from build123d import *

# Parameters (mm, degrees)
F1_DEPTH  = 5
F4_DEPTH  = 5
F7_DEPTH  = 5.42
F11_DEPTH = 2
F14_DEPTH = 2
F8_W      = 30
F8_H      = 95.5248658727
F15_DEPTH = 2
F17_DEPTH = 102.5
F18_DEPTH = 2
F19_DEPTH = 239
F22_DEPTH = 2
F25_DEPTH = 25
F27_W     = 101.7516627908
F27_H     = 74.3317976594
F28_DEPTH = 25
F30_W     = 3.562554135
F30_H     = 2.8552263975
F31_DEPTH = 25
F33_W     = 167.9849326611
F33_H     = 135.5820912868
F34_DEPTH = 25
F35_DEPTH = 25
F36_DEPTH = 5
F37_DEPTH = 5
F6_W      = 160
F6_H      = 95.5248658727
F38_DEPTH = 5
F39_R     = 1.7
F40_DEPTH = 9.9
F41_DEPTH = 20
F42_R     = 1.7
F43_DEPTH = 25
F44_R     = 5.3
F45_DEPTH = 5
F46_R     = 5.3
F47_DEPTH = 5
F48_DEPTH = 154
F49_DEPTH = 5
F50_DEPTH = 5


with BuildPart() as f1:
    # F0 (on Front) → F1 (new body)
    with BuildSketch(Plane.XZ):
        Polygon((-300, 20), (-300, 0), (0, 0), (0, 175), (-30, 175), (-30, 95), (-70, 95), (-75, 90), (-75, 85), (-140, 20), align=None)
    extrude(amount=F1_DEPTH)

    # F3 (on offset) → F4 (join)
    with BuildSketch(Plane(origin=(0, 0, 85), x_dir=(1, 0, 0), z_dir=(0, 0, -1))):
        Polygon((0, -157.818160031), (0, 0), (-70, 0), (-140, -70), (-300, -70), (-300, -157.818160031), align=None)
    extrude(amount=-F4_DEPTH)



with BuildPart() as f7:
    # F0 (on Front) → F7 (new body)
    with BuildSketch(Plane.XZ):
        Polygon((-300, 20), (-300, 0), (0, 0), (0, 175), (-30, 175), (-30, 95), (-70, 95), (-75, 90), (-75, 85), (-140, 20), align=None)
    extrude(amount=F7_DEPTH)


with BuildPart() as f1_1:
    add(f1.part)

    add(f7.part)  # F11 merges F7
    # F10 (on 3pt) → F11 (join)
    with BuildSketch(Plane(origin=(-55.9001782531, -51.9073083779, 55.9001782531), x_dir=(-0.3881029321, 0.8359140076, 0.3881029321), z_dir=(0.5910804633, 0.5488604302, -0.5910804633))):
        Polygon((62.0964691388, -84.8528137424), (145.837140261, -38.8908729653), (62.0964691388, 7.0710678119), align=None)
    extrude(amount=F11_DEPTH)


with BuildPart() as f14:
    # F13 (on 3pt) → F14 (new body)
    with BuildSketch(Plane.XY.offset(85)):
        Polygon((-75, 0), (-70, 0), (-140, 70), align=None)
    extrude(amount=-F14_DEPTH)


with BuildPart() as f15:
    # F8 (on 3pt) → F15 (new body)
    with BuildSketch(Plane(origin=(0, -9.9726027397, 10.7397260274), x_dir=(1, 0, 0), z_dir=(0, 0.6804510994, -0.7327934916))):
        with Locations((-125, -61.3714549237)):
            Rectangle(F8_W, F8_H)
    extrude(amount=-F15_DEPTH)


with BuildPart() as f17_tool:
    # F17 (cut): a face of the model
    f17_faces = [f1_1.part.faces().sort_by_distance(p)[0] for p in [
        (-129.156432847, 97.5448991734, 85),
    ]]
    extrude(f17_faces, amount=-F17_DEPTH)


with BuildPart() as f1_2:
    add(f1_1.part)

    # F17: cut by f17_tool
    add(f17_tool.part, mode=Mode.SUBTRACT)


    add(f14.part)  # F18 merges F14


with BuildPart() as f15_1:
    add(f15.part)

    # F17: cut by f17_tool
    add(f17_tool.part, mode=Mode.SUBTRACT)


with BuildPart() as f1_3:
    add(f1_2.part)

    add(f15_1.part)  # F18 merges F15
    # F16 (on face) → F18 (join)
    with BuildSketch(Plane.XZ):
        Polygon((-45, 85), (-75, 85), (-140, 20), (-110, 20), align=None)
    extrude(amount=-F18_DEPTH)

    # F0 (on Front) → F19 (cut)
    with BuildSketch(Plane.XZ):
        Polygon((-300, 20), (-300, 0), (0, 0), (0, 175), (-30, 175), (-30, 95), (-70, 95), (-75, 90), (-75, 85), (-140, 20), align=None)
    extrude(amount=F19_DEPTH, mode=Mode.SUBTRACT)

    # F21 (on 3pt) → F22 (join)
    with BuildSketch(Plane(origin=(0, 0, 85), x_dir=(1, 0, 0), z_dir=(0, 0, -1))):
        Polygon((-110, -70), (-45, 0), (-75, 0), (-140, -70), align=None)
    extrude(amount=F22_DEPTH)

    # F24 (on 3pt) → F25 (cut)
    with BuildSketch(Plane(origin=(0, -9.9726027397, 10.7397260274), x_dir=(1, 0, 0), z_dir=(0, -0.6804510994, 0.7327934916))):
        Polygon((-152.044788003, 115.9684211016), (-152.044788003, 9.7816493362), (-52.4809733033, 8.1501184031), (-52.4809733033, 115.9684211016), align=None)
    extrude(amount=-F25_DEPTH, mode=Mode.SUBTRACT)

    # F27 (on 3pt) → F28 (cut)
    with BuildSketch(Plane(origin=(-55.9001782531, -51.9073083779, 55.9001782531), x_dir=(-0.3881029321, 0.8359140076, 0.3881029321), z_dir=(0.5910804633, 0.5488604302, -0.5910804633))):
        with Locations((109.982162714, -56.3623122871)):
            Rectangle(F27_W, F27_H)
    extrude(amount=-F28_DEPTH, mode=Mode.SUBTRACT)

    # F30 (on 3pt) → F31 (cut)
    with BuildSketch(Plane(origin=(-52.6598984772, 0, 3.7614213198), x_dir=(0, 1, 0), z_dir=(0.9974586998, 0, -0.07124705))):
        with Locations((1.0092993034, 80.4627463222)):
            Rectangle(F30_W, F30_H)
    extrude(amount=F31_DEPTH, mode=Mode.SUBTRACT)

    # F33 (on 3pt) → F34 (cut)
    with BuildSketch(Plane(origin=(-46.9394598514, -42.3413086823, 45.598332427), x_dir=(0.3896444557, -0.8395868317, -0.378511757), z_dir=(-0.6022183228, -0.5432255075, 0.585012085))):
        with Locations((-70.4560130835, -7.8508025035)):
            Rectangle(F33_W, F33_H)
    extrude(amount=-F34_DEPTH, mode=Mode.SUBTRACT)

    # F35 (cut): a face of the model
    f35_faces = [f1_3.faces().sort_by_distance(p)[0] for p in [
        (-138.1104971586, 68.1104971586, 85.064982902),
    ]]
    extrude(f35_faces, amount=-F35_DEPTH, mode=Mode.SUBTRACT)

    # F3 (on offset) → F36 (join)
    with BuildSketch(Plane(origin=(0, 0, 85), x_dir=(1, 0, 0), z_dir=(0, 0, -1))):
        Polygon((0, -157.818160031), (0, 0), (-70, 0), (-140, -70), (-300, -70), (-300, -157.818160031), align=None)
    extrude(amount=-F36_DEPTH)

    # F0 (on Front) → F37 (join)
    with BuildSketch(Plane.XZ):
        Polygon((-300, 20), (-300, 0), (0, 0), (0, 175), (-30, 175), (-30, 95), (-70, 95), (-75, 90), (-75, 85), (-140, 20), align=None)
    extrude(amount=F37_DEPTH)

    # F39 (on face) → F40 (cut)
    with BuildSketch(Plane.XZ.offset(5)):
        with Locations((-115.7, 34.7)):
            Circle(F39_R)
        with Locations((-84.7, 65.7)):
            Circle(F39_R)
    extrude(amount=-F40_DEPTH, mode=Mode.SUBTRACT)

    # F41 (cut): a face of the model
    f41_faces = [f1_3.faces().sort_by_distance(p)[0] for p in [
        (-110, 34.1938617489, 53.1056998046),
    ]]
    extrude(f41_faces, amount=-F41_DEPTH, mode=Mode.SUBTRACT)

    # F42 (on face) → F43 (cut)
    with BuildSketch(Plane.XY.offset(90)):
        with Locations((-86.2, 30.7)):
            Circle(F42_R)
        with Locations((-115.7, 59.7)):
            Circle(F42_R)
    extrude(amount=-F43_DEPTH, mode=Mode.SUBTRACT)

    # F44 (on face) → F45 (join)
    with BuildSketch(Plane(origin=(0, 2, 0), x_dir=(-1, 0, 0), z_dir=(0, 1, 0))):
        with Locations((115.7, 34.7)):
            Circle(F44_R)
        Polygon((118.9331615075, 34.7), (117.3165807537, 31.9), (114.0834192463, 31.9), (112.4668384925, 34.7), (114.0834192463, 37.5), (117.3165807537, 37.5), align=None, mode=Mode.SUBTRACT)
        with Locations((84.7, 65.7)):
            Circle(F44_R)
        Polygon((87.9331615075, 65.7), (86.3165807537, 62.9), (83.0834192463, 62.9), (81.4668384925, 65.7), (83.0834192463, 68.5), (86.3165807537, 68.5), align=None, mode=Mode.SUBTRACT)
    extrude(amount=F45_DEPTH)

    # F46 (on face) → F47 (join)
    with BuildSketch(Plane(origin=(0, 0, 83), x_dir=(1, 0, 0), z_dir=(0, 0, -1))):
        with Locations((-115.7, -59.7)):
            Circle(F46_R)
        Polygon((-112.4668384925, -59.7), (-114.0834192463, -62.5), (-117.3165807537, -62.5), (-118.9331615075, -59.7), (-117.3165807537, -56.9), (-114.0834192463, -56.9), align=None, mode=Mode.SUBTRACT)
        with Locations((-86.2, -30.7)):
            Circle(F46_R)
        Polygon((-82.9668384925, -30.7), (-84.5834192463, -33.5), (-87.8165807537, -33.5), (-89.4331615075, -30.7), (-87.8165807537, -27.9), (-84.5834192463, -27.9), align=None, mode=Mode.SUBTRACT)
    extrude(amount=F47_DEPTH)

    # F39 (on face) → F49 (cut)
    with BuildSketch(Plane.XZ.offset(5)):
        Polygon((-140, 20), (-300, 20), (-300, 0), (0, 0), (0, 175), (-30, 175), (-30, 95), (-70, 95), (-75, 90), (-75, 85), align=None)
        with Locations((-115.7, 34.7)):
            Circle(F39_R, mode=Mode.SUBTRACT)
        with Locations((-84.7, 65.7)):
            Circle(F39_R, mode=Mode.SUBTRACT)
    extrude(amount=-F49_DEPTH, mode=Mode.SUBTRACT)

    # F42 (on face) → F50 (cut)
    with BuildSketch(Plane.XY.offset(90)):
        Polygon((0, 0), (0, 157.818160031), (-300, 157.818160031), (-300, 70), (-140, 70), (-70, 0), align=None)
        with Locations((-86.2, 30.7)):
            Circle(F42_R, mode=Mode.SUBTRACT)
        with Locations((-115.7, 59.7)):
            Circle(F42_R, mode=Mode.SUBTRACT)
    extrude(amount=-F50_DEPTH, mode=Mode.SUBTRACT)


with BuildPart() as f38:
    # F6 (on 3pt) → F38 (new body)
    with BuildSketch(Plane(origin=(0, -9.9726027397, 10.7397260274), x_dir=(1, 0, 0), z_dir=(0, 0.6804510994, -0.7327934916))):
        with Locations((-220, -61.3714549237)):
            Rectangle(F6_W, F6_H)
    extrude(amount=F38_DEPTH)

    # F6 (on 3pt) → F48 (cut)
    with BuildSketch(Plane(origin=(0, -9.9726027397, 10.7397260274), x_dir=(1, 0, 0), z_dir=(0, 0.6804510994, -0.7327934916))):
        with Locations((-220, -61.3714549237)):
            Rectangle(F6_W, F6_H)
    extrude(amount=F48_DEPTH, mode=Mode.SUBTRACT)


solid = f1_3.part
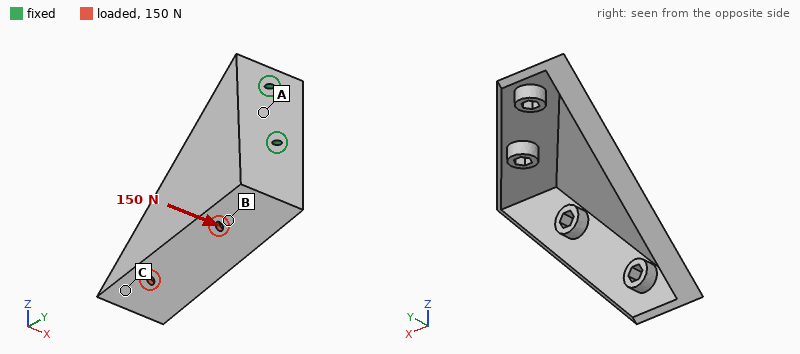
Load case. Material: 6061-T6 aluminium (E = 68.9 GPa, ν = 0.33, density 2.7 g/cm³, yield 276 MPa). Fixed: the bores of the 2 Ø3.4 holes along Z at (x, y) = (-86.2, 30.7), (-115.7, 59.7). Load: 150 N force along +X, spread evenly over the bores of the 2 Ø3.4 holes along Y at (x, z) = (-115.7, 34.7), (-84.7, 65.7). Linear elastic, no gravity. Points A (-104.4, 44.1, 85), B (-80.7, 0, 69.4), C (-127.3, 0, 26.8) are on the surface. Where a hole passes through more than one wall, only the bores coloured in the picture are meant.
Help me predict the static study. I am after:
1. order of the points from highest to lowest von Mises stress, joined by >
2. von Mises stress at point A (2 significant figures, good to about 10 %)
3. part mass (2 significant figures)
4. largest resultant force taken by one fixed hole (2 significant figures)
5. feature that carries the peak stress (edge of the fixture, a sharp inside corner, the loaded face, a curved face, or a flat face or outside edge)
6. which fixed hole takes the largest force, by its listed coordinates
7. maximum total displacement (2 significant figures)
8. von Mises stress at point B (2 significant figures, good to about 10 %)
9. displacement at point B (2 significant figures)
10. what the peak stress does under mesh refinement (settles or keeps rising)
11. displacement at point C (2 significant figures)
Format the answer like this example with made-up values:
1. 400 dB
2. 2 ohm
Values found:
1. A > B > C
2. 23 MPa
3. 45 g
4. 220 N
5. edge of the fixture
6. (-86.2, 30.7)
7. 1.5 mm
8. 16 MPa
9. 0.30 mm
10. keeps rising
11. 1.3 mm
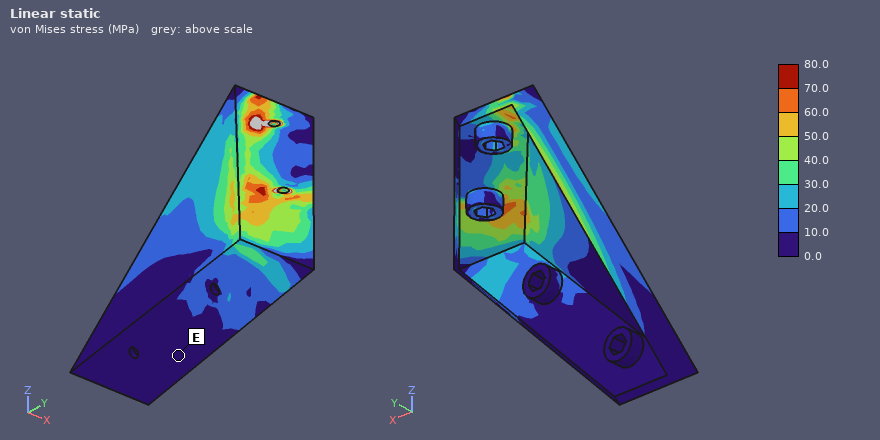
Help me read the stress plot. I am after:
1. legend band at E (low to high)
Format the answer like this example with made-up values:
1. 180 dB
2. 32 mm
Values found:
1. 0.0 to 10.0 MPa
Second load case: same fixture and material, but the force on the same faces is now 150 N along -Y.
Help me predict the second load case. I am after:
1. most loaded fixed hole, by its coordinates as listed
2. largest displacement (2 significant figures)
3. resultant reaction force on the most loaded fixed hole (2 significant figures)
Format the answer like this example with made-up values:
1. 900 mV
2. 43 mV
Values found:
1. (-86.2, 30.7)
2. 1.5 mm
3. 140 N
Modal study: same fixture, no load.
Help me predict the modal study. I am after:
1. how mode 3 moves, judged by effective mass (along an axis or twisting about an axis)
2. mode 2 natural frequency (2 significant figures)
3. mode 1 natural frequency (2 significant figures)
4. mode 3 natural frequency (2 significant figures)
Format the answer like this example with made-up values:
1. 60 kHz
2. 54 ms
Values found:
1. along Z
2. 1300 Hz
3. 340 Hz
4. 1700 Hz
